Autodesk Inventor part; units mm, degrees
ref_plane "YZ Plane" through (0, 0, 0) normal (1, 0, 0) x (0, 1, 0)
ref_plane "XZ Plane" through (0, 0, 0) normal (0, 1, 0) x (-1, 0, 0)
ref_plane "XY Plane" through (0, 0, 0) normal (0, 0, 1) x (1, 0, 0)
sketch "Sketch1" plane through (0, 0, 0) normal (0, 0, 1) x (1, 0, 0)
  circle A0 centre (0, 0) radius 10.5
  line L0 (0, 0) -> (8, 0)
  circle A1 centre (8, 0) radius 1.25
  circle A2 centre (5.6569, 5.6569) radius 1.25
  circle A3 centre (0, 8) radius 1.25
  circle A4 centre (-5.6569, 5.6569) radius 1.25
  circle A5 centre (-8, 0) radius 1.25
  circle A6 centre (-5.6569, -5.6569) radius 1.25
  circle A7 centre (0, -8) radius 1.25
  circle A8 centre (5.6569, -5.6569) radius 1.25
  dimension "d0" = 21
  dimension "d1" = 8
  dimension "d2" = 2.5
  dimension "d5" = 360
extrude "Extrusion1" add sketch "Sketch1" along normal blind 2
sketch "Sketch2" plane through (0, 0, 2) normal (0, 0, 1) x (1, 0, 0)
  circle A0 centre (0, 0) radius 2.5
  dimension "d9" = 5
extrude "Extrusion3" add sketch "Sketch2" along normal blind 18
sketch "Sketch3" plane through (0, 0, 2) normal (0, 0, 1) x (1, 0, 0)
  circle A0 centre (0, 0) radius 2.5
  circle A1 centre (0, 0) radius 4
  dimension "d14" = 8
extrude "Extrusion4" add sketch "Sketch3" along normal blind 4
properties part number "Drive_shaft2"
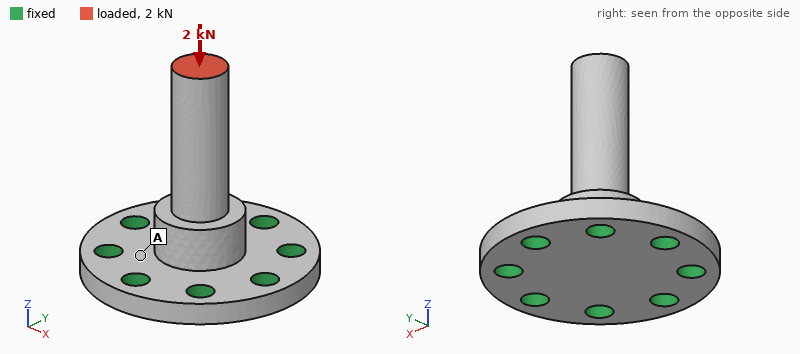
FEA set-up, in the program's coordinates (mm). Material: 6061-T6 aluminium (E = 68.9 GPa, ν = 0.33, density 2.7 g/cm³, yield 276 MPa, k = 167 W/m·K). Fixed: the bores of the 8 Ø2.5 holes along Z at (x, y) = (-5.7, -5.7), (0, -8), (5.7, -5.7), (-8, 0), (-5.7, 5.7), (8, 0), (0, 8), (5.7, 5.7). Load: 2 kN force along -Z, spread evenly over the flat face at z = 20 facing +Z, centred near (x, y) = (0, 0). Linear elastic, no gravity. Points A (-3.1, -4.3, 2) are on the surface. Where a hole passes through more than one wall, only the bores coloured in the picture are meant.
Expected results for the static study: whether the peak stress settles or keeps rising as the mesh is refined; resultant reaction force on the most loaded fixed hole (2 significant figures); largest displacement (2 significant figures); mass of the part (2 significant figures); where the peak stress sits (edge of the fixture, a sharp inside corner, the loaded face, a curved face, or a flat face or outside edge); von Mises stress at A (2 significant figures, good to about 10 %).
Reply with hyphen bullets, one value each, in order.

- keeps rising
- 280 N
- 36 µm
- 2.9 g
- edge of the fixture
- 33 MPa
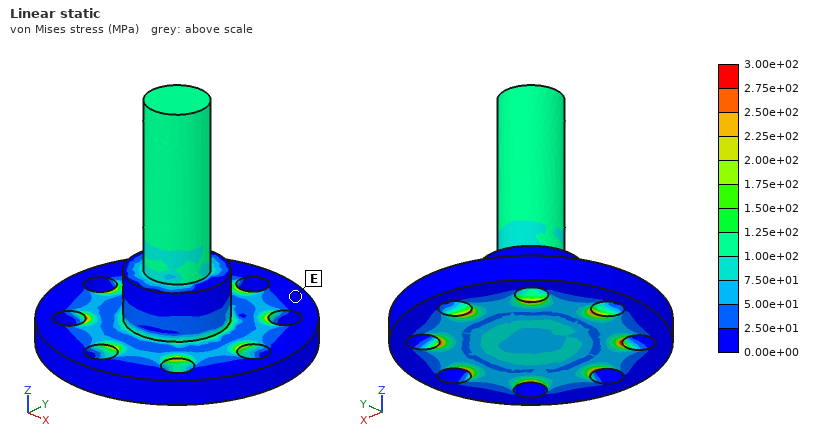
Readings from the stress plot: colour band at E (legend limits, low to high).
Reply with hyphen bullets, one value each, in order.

- 0.00e+00 to 2.50e+01 MPa
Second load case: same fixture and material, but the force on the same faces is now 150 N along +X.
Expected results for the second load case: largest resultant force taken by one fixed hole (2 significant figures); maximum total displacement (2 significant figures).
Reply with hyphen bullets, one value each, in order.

- 130 N
- 0.11 mm
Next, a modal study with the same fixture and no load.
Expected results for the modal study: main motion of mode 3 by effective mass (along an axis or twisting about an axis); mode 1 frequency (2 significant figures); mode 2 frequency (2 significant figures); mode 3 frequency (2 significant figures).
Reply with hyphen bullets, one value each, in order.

- along Z
- 12 kHz
- 12 kHz
- 45 kHz
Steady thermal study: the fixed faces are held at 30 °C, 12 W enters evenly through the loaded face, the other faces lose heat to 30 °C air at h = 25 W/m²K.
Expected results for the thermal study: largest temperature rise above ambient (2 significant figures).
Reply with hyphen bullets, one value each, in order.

- 63 K
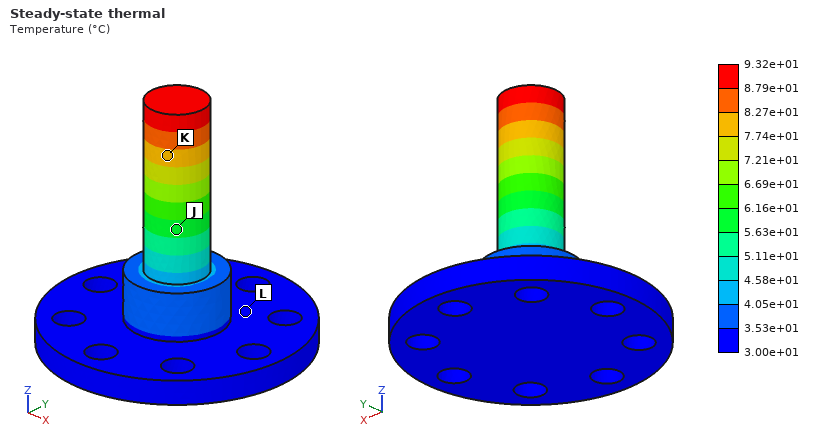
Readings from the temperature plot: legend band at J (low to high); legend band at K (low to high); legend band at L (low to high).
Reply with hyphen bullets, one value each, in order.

- 5.63e+01 to 6.16e+01 °C
- 7.74e+01 to 8.27e+01 °C
- 3.00e+01 to 3.53e+01 °C
